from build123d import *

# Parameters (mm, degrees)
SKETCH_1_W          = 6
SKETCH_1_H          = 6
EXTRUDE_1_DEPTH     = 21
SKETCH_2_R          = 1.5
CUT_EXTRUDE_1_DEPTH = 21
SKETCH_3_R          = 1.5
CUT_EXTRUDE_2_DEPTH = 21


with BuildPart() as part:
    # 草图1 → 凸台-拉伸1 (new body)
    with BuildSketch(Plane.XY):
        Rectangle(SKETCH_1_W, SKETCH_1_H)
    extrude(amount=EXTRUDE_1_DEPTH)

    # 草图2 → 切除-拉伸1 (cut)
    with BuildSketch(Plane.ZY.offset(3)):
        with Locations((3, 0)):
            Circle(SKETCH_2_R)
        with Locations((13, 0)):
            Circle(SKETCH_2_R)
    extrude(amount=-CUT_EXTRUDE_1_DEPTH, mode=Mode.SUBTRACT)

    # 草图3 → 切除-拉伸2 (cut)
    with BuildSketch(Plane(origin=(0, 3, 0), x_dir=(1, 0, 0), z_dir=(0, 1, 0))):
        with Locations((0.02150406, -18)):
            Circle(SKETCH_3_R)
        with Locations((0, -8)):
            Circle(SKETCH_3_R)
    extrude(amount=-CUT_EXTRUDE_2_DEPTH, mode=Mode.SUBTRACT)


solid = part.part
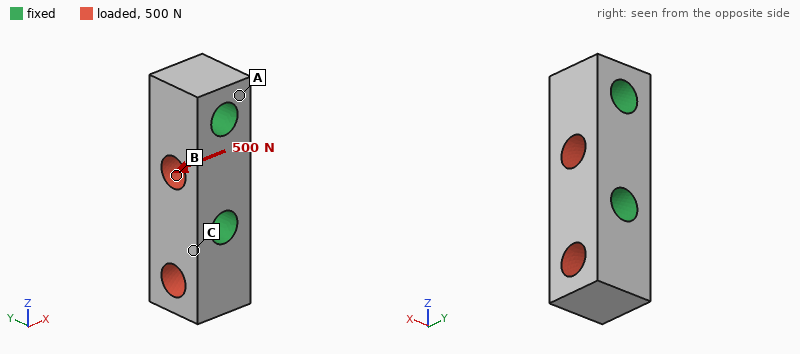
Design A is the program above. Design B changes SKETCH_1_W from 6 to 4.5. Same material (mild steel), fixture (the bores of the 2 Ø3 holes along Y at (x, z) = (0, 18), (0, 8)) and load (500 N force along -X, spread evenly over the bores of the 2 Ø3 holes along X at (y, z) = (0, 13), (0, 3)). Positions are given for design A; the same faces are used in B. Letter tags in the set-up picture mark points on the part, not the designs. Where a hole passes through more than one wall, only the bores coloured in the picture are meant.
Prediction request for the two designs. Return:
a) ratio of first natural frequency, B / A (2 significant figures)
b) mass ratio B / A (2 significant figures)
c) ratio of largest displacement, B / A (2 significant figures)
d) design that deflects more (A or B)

0.93
0.71
1.6
B
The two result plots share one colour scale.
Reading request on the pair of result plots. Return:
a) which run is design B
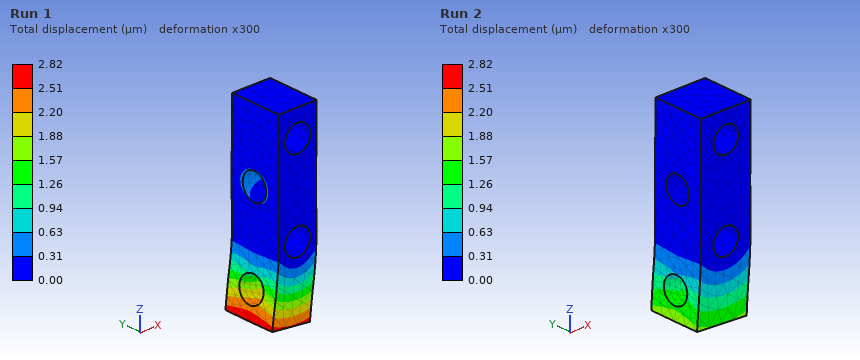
Run 1
